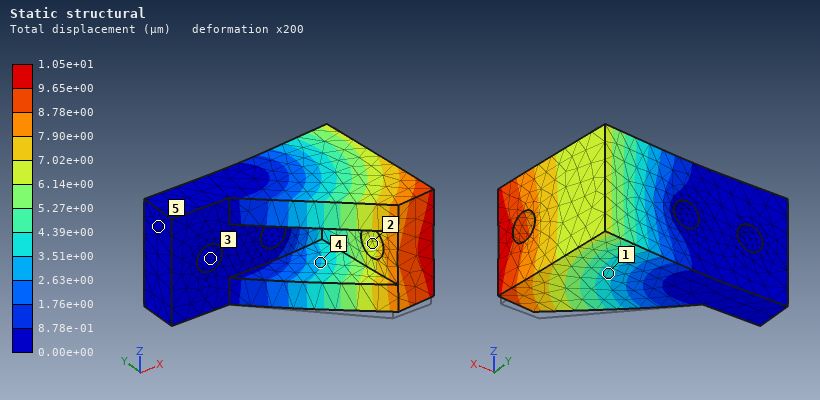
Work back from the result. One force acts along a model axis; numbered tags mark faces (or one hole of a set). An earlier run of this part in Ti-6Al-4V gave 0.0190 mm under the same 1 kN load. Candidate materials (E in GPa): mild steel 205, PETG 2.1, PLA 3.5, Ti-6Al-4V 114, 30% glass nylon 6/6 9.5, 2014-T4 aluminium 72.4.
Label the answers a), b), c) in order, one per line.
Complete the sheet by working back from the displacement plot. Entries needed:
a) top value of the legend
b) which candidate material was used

a) 1.05e+01 µm
b) mild steel
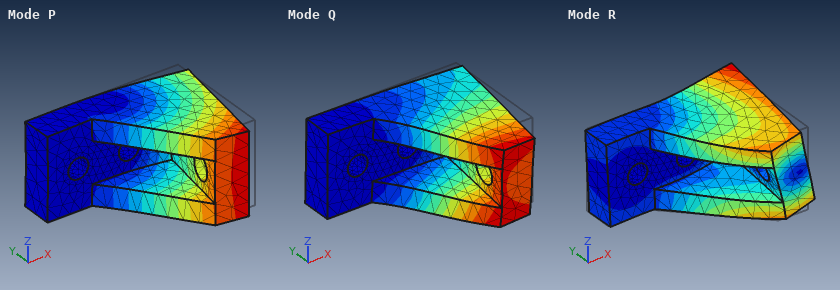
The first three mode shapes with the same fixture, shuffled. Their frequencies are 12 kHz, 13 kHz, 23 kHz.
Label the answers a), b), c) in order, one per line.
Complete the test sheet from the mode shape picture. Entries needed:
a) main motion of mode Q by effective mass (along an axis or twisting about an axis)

a) along Z
